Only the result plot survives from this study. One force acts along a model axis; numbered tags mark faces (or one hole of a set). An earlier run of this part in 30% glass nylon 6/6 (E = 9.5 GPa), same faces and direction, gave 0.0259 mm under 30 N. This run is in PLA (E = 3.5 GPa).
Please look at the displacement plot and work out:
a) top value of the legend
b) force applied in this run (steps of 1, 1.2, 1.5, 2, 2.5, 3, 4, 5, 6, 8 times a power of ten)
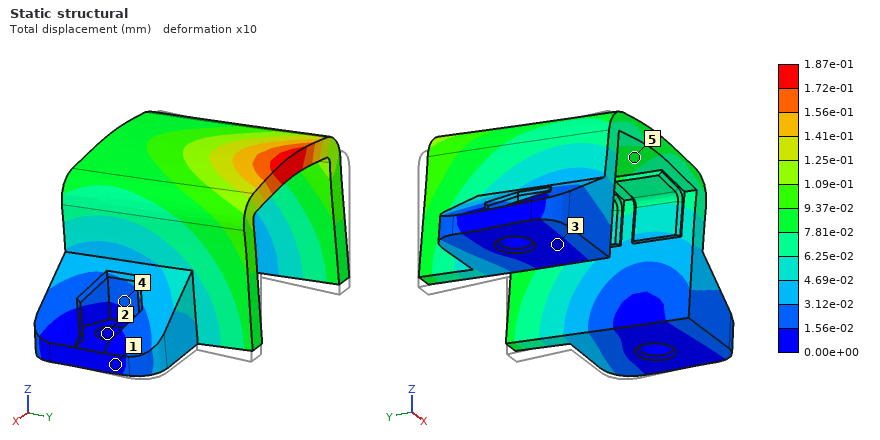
1.87e-01 mm
80 N
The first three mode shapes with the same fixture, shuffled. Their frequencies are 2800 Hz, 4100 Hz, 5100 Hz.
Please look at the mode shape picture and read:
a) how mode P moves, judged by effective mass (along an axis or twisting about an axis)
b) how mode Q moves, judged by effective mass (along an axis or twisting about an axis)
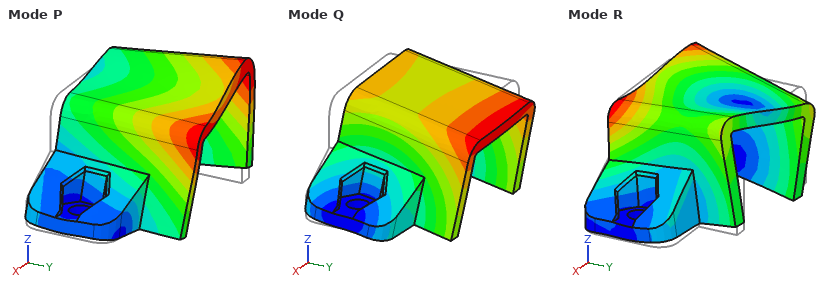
along X
along Y
